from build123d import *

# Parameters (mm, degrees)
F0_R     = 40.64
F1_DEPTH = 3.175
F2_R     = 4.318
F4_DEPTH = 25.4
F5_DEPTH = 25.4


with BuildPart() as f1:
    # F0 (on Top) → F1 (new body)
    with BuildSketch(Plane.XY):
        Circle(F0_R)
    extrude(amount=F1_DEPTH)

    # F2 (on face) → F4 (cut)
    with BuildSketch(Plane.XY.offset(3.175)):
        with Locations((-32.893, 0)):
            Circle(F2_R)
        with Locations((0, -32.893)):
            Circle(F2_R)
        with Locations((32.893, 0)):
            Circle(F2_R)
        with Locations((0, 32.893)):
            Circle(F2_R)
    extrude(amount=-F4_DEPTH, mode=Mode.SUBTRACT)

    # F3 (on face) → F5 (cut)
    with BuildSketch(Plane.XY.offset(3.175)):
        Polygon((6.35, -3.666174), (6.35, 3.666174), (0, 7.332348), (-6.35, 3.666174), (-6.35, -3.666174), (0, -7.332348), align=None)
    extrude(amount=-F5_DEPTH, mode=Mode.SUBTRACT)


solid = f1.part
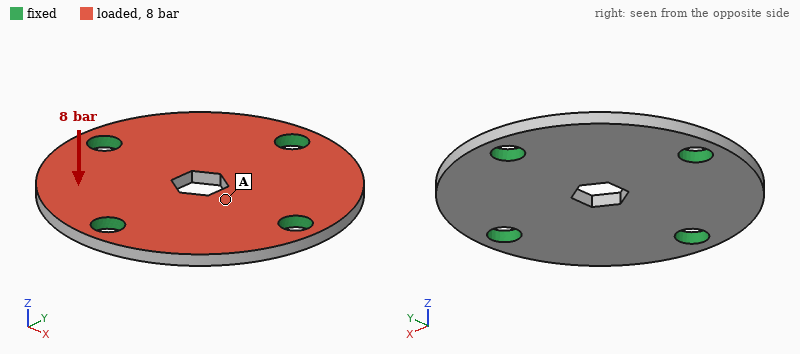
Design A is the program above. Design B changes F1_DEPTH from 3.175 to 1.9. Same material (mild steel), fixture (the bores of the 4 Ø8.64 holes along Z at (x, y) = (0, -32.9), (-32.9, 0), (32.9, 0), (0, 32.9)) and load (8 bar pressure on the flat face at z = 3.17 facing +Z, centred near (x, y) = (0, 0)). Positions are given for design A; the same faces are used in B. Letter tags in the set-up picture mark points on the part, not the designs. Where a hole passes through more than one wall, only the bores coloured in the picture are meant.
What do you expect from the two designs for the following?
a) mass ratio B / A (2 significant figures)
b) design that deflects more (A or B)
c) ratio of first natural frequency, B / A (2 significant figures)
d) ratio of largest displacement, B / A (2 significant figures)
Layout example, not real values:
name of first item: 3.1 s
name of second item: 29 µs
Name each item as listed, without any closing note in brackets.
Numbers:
mass ratio B / A: 0.60
design that deflects more: B
ratio of first natural frequency, B / A: 0.62
ratio of largest displacement, B / A: 4.4
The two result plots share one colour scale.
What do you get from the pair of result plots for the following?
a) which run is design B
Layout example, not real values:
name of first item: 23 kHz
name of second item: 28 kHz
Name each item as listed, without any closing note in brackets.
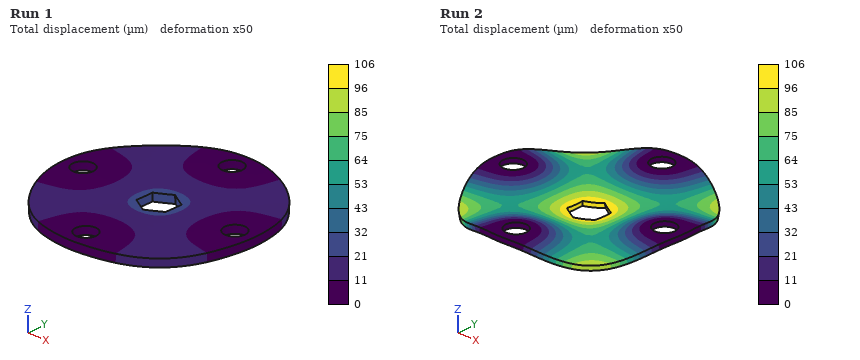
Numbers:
which run is design B: Run 2
